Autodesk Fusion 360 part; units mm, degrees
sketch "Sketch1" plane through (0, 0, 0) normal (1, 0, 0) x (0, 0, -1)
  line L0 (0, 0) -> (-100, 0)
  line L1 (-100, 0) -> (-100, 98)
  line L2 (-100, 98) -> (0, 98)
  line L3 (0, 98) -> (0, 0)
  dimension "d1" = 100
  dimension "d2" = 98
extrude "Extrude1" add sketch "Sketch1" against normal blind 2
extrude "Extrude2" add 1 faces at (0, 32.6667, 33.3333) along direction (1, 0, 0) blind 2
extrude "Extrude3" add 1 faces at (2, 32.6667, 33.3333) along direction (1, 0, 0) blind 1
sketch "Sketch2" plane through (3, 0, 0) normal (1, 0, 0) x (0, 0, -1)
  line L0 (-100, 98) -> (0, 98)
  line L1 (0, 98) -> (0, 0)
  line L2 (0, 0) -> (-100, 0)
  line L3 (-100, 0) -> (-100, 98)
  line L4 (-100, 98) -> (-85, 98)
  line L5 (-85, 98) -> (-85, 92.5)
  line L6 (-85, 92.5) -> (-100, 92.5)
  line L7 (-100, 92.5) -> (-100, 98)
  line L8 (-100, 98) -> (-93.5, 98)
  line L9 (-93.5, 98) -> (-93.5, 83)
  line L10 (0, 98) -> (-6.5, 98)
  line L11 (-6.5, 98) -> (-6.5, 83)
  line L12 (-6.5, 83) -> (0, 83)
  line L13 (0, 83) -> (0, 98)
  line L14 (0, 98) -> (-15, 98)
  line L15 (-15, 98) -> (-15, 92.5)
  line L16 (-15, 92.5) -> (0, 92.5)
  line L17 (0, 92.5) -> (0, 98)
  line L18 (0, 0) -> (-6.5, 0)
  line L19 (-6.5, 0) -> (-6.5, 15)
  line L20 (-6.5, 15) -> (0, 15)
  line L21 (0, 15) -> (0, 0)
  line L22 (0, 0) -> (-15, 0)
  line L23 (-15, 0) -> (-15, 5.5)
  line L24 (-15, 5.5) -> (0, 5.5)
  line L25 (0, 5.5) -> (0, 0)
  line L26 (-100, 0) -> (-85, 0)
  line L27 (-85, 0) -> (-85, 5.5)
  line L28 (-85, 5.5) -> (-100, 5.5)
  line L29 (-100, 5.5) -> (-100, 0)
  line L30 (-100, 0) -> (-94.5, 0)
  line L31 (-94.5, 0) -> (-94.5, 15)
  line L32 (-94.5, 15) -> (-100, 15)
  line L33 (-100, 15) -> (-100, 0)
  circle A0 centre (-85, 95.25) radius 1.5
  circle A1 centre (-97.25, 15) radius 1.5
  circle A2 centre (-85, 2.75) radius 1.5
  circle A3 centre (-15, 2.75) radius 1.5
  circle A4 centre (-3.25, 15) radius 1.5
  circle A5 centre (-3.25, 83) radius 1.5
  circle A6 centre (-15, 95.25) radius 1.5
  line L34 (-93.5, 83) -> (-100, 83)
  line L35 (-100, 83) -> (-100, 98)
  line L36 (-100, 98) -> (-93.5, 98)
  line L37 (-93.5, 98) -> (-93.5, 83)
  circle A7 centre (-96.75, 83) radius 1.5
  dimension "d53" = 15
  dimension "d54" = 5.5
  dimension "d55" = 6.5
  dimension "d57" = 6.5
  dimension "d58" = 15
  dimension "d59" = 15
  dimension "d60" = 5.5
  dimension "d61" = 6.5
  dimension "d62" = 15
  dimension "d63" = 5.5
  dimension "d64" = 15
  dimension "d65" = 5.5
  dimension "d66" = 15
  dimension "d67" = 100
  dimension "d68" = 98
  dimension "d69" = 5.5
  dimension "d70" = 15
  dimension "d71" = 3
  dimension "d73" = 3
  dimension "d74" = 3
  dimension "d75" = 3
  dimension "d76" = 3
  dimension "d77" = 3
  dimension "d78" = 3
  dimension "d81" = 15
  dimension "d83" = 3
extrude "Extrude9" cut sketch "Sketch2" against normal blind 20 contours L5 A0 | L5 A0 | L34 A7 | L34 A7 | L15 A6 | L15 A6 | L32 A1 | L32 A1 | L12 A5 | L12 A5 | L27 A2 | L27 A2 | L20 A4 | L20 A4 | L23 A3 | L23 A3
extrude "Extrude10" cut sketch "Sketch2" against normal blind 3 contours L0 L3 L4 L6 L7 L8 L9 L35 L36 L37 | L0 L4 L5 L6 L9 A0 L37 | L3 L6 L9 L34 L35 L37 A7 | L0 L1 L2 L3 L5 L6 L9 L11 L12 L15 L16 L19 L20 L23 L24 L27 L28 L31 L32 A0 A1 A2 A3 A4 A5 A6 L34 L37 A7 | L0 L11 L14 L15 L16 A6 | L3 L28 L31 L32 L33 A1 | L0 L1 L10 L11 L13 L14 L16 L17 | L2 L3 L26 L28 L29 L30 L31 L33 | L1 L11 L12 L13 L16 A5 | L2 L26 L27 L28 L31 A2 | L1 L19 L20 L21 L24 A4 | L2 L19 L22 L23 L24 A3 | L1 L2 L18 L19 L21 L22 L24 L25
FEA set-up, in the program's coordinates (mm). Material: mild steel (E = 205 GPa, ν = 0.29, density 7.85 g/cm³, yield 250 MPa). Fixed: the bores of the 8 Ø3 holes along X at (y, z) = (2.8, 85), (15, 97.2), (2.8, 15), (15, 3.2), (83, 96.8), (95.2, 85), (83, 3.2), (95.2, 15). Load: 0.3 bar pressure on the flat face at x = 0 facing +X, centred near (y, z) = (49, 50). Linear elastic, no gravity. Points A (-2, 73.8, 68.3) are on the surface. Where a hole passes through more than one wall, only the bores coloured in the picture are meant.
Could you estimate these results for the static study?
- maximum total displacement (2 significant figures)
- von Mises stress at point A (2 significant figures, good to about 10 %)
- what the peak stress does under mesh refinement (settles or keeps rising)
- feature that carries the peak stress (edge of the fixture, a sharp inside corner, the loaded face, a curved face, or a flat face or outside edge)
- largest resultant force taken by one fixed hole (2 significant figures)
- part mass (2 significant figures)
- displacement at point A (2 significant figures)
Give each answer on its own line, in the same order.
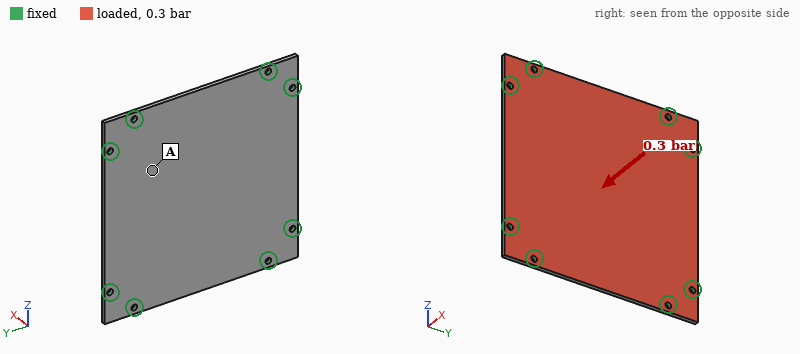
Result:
59 µm
8.0 MPa
keeps rising
edge of the fixture
38 N
150 g
35 µm
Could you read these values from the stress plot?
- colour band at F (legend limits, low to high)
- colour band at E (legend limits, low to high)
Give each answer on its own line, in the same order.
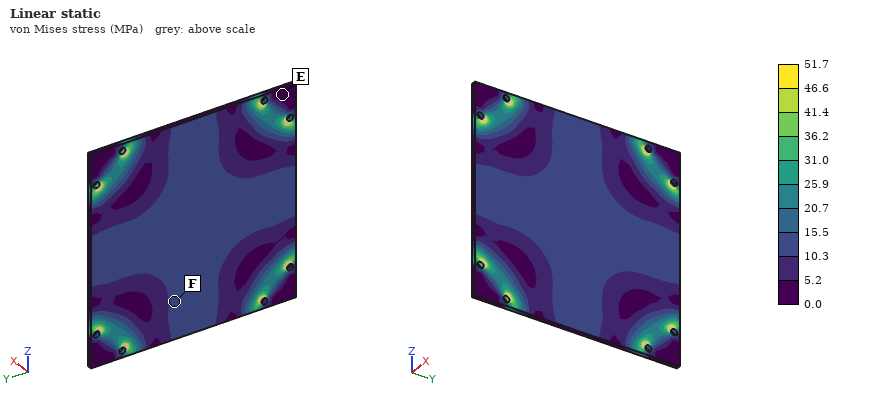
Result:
10.3 to 15.5 MPa
0.0 to 5.2 MPa
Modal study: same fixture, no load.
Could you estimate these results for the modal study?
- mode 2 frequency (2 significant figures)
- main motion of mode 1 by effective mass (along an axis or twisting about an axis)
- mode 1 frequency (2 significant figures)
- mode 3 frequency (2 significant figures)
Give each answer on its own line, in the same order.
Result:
2100 Hz
along X
1100 Hz
2100 Hz
